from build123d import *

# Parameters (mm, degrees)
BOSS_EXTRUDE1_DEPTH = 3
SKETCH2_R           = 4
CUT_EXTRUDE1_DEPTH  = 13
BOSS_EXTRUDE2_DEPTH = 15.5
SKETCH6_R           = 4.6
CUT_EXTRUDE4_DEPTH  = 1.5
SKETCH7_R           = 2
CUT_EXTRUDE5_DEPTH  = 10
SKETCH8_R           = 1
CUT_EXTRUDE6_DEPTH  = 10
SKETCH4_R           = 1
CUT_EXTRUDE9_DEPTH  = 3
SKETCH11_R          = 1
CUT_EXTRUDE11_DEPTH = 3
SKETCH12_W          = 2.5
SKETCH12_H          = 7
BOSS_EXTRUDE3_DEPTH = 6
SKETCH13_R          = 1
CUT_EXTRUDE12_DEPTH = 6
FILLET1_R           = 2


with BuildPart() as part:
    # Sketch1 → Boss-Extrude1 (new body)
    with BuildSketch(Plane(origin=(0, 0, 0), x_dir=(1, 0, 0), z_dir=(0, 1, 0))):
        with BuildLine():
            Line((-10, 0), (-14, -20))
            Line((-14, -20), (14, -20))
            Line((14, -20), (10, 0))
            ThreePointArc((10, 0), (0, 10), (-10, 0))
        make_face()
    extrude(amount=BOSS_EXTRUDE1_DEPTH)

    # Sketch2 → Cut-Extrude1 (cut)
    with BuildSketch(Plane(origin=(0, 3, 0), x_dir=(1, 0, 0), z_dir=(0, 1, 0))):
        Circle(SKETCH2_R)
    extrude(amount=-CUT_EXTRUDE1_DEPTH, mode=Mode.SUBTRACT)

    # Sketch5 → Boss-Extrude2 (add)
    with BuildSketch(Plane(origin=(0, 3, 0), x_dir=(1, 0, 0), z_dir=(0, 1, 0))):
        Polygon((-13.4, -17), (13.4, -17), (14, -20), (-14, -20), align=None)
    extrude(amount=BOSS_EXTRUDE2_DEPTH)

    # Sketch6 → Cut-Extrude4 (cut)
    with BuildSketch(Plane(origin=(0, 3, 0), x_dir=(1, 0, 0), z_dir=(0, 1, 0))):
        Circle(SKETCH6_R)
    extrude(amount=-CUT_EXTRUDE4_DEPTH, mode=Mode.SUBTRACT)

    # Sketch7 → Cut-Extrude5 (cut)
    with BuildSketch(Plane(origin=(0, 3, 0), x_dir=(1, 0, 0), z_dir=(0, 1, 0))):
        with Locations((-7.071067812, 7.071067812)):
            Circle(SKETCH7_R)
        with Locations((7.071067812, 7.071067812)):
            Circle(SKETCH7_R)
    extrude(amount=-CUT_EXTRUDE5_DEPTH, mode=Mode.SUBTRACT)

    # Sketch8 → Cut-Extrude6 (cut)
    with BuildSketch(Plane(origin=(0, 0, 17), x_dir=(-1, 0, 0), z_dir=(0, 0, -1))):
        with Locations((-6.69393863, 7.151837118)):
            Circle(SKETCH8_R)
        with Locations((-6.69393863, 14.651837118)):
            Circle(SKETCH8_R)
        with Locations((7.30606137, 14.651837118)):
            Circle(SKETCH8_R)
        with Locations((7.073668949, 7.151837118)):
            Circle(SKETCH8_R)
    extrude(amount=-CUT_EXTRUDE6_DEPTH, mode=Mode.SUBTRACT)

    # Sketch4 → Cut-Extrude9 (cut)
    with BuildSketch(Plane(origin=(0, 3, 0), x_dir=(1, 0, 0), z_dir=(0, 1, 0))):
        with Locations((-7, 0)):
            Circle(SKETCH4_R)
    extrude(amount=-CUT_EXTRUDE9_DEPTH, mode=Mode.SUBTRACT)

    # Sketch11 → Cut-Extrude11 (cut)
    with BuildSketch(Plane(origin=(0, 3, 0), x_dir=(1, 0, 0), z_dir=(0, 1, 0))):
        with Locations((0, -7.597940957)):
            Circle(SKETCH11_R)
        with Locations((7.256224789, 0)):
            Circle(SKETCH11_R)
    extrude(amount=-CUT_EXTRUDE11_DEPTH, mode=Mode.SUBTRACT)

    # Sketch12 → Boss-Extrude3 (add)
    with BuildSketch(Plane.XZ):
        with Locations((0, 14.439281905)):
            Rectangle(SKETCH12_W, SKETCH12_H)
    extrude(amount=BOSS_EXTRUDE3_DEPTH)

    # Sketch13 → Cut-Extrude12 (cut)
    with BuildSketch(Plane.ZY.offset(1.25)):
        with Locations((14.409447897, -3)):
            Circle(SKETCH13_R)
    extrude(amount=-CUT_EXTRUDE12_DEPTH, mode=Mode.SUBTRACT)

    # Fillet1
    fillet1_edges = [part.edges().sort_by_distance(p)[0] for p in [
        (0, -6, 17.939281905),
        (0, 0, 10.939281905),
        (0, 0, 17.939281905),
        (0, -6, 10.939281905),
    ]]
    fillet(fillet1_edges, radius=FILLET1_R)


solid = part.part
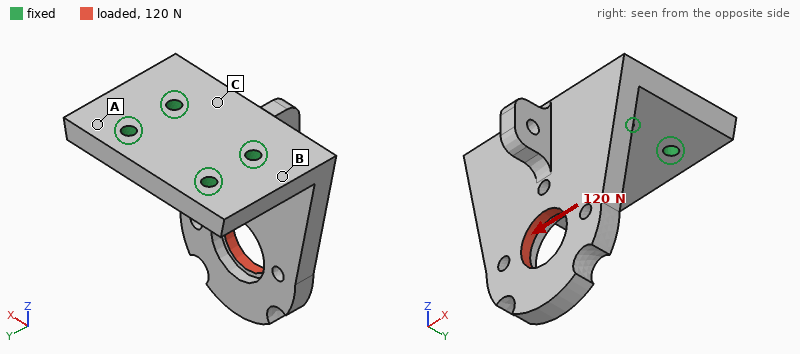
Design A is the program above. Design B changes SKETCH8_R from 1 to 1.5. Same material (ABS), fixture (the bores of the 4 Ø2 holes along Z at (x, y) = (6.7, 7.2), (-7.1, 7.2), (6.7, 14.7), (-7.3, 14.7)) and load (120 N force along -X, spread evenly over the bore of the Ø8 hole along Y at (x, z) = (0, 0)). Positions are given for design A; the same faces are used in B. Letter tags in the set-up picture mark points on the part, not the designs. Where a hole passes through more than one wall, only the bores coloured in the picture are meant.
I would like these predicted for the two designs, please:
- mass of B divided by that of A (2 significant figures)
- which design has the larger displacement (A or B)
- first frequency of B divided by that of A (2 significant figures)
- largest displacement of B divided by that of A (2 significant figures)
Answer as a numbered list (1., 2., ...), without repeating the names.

1. 0.98
2. A
3. 1.0
4. 0.82
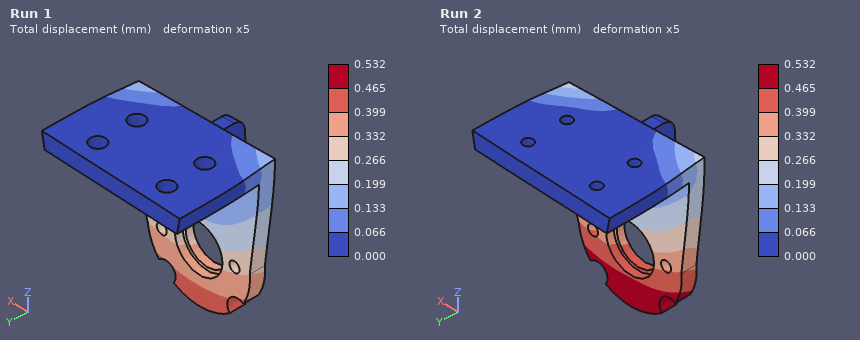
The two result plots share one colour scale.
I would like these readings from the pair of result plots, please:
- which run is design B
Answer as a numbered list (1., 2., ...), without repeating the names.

1. Run 1
